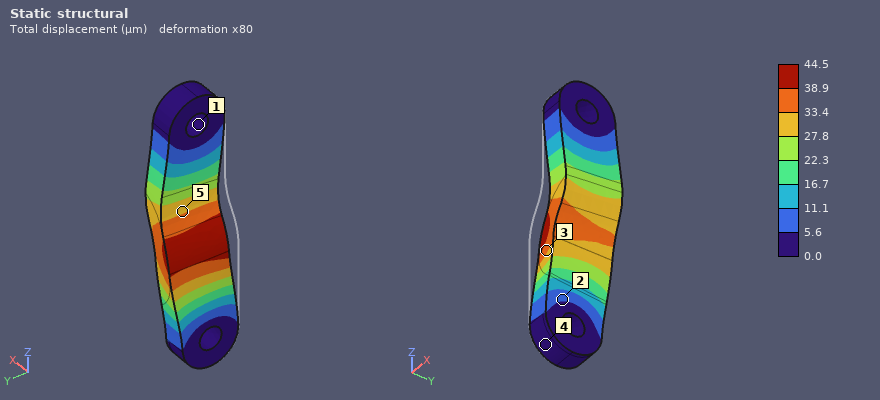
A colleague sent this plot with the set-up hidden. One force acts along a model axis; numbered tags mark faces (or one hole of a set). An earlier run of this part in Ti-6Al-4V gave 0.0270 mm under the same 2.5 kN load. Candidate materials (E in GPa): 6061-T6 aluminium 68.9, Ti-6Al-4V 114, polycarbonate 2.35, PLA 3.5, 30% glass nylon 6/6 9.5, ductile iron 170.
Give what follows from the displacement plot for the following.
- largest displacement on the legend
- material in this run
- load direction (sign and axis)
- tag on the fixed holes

44.5 µm
6061-T6 aluminium
+Y
1
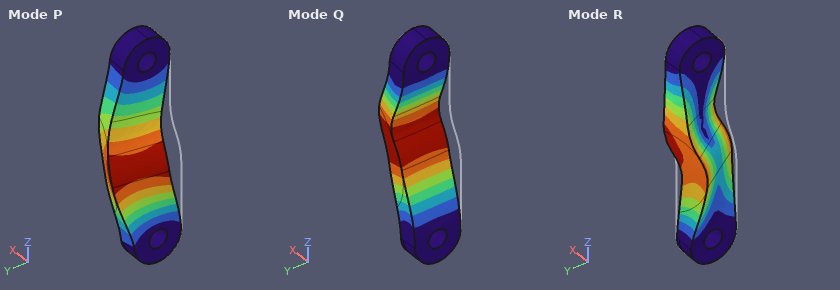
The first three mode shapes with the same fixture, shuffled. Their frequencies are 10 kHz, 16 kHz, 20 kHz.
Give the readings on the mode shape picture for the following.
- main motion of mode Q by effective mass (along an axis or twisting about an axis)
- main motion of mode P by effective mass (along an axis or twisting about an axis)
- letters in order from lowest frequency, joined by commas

along X
along Y
Q, P, R
